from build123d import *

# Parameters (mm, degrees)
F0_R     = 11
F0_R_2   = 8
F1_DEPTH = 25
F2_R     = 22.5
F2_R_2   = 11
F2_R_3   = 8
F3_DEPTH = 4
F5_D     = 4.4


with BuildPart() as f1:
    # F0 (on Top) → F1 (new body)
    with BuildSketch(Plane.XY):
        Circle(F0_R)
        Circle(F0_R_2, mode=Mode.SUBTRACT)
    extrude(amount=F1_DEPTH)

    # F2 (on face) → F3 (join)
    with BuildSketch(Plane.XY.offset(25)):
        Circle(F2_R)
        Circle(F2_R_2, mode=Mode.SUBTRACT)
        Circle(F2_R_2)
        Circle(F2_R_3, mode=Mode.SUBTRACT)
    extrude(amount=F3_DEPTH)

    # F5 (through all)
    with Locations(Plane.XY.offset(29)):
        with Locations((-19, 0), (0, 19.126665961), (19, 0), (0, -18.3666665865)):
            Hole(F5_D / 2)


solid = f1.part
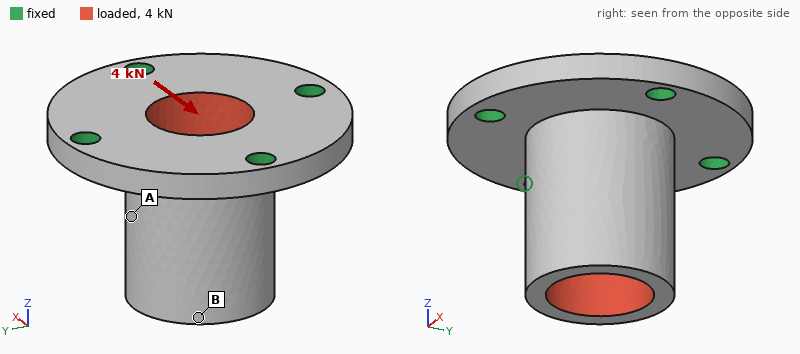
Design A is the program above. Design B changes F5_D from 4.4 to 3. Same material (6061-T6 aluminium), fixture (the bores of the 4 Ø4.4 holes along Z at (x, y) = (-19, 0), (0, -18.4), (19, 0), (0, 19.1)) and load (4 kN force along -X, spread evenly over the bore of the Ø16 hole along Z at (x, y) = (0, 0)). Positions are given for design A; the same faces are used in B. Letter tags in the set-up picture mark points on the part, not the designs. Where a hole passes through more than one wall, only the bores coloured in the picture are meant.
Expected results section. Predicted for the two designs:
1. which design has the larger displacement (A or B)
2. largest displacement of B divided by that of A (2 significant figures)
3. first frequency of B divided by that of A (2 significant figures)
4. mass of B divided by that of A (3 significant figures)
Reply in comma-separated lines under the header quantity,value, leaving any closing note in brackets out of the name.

quantity,value
which design has the larger displacement,B
largest displacement of B divided by that of A,1.1
first frequency of B divided by that of A,0.94
mass of B divided by that of A,1.01
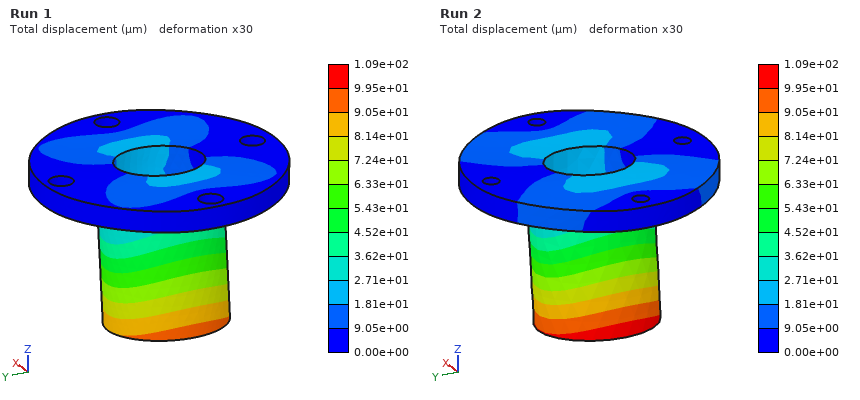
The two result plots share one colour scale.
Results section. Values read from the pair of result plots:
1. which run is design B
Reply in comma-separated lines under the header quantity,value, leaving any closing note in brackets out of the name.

quantity,value
which run is design B,Run 2
